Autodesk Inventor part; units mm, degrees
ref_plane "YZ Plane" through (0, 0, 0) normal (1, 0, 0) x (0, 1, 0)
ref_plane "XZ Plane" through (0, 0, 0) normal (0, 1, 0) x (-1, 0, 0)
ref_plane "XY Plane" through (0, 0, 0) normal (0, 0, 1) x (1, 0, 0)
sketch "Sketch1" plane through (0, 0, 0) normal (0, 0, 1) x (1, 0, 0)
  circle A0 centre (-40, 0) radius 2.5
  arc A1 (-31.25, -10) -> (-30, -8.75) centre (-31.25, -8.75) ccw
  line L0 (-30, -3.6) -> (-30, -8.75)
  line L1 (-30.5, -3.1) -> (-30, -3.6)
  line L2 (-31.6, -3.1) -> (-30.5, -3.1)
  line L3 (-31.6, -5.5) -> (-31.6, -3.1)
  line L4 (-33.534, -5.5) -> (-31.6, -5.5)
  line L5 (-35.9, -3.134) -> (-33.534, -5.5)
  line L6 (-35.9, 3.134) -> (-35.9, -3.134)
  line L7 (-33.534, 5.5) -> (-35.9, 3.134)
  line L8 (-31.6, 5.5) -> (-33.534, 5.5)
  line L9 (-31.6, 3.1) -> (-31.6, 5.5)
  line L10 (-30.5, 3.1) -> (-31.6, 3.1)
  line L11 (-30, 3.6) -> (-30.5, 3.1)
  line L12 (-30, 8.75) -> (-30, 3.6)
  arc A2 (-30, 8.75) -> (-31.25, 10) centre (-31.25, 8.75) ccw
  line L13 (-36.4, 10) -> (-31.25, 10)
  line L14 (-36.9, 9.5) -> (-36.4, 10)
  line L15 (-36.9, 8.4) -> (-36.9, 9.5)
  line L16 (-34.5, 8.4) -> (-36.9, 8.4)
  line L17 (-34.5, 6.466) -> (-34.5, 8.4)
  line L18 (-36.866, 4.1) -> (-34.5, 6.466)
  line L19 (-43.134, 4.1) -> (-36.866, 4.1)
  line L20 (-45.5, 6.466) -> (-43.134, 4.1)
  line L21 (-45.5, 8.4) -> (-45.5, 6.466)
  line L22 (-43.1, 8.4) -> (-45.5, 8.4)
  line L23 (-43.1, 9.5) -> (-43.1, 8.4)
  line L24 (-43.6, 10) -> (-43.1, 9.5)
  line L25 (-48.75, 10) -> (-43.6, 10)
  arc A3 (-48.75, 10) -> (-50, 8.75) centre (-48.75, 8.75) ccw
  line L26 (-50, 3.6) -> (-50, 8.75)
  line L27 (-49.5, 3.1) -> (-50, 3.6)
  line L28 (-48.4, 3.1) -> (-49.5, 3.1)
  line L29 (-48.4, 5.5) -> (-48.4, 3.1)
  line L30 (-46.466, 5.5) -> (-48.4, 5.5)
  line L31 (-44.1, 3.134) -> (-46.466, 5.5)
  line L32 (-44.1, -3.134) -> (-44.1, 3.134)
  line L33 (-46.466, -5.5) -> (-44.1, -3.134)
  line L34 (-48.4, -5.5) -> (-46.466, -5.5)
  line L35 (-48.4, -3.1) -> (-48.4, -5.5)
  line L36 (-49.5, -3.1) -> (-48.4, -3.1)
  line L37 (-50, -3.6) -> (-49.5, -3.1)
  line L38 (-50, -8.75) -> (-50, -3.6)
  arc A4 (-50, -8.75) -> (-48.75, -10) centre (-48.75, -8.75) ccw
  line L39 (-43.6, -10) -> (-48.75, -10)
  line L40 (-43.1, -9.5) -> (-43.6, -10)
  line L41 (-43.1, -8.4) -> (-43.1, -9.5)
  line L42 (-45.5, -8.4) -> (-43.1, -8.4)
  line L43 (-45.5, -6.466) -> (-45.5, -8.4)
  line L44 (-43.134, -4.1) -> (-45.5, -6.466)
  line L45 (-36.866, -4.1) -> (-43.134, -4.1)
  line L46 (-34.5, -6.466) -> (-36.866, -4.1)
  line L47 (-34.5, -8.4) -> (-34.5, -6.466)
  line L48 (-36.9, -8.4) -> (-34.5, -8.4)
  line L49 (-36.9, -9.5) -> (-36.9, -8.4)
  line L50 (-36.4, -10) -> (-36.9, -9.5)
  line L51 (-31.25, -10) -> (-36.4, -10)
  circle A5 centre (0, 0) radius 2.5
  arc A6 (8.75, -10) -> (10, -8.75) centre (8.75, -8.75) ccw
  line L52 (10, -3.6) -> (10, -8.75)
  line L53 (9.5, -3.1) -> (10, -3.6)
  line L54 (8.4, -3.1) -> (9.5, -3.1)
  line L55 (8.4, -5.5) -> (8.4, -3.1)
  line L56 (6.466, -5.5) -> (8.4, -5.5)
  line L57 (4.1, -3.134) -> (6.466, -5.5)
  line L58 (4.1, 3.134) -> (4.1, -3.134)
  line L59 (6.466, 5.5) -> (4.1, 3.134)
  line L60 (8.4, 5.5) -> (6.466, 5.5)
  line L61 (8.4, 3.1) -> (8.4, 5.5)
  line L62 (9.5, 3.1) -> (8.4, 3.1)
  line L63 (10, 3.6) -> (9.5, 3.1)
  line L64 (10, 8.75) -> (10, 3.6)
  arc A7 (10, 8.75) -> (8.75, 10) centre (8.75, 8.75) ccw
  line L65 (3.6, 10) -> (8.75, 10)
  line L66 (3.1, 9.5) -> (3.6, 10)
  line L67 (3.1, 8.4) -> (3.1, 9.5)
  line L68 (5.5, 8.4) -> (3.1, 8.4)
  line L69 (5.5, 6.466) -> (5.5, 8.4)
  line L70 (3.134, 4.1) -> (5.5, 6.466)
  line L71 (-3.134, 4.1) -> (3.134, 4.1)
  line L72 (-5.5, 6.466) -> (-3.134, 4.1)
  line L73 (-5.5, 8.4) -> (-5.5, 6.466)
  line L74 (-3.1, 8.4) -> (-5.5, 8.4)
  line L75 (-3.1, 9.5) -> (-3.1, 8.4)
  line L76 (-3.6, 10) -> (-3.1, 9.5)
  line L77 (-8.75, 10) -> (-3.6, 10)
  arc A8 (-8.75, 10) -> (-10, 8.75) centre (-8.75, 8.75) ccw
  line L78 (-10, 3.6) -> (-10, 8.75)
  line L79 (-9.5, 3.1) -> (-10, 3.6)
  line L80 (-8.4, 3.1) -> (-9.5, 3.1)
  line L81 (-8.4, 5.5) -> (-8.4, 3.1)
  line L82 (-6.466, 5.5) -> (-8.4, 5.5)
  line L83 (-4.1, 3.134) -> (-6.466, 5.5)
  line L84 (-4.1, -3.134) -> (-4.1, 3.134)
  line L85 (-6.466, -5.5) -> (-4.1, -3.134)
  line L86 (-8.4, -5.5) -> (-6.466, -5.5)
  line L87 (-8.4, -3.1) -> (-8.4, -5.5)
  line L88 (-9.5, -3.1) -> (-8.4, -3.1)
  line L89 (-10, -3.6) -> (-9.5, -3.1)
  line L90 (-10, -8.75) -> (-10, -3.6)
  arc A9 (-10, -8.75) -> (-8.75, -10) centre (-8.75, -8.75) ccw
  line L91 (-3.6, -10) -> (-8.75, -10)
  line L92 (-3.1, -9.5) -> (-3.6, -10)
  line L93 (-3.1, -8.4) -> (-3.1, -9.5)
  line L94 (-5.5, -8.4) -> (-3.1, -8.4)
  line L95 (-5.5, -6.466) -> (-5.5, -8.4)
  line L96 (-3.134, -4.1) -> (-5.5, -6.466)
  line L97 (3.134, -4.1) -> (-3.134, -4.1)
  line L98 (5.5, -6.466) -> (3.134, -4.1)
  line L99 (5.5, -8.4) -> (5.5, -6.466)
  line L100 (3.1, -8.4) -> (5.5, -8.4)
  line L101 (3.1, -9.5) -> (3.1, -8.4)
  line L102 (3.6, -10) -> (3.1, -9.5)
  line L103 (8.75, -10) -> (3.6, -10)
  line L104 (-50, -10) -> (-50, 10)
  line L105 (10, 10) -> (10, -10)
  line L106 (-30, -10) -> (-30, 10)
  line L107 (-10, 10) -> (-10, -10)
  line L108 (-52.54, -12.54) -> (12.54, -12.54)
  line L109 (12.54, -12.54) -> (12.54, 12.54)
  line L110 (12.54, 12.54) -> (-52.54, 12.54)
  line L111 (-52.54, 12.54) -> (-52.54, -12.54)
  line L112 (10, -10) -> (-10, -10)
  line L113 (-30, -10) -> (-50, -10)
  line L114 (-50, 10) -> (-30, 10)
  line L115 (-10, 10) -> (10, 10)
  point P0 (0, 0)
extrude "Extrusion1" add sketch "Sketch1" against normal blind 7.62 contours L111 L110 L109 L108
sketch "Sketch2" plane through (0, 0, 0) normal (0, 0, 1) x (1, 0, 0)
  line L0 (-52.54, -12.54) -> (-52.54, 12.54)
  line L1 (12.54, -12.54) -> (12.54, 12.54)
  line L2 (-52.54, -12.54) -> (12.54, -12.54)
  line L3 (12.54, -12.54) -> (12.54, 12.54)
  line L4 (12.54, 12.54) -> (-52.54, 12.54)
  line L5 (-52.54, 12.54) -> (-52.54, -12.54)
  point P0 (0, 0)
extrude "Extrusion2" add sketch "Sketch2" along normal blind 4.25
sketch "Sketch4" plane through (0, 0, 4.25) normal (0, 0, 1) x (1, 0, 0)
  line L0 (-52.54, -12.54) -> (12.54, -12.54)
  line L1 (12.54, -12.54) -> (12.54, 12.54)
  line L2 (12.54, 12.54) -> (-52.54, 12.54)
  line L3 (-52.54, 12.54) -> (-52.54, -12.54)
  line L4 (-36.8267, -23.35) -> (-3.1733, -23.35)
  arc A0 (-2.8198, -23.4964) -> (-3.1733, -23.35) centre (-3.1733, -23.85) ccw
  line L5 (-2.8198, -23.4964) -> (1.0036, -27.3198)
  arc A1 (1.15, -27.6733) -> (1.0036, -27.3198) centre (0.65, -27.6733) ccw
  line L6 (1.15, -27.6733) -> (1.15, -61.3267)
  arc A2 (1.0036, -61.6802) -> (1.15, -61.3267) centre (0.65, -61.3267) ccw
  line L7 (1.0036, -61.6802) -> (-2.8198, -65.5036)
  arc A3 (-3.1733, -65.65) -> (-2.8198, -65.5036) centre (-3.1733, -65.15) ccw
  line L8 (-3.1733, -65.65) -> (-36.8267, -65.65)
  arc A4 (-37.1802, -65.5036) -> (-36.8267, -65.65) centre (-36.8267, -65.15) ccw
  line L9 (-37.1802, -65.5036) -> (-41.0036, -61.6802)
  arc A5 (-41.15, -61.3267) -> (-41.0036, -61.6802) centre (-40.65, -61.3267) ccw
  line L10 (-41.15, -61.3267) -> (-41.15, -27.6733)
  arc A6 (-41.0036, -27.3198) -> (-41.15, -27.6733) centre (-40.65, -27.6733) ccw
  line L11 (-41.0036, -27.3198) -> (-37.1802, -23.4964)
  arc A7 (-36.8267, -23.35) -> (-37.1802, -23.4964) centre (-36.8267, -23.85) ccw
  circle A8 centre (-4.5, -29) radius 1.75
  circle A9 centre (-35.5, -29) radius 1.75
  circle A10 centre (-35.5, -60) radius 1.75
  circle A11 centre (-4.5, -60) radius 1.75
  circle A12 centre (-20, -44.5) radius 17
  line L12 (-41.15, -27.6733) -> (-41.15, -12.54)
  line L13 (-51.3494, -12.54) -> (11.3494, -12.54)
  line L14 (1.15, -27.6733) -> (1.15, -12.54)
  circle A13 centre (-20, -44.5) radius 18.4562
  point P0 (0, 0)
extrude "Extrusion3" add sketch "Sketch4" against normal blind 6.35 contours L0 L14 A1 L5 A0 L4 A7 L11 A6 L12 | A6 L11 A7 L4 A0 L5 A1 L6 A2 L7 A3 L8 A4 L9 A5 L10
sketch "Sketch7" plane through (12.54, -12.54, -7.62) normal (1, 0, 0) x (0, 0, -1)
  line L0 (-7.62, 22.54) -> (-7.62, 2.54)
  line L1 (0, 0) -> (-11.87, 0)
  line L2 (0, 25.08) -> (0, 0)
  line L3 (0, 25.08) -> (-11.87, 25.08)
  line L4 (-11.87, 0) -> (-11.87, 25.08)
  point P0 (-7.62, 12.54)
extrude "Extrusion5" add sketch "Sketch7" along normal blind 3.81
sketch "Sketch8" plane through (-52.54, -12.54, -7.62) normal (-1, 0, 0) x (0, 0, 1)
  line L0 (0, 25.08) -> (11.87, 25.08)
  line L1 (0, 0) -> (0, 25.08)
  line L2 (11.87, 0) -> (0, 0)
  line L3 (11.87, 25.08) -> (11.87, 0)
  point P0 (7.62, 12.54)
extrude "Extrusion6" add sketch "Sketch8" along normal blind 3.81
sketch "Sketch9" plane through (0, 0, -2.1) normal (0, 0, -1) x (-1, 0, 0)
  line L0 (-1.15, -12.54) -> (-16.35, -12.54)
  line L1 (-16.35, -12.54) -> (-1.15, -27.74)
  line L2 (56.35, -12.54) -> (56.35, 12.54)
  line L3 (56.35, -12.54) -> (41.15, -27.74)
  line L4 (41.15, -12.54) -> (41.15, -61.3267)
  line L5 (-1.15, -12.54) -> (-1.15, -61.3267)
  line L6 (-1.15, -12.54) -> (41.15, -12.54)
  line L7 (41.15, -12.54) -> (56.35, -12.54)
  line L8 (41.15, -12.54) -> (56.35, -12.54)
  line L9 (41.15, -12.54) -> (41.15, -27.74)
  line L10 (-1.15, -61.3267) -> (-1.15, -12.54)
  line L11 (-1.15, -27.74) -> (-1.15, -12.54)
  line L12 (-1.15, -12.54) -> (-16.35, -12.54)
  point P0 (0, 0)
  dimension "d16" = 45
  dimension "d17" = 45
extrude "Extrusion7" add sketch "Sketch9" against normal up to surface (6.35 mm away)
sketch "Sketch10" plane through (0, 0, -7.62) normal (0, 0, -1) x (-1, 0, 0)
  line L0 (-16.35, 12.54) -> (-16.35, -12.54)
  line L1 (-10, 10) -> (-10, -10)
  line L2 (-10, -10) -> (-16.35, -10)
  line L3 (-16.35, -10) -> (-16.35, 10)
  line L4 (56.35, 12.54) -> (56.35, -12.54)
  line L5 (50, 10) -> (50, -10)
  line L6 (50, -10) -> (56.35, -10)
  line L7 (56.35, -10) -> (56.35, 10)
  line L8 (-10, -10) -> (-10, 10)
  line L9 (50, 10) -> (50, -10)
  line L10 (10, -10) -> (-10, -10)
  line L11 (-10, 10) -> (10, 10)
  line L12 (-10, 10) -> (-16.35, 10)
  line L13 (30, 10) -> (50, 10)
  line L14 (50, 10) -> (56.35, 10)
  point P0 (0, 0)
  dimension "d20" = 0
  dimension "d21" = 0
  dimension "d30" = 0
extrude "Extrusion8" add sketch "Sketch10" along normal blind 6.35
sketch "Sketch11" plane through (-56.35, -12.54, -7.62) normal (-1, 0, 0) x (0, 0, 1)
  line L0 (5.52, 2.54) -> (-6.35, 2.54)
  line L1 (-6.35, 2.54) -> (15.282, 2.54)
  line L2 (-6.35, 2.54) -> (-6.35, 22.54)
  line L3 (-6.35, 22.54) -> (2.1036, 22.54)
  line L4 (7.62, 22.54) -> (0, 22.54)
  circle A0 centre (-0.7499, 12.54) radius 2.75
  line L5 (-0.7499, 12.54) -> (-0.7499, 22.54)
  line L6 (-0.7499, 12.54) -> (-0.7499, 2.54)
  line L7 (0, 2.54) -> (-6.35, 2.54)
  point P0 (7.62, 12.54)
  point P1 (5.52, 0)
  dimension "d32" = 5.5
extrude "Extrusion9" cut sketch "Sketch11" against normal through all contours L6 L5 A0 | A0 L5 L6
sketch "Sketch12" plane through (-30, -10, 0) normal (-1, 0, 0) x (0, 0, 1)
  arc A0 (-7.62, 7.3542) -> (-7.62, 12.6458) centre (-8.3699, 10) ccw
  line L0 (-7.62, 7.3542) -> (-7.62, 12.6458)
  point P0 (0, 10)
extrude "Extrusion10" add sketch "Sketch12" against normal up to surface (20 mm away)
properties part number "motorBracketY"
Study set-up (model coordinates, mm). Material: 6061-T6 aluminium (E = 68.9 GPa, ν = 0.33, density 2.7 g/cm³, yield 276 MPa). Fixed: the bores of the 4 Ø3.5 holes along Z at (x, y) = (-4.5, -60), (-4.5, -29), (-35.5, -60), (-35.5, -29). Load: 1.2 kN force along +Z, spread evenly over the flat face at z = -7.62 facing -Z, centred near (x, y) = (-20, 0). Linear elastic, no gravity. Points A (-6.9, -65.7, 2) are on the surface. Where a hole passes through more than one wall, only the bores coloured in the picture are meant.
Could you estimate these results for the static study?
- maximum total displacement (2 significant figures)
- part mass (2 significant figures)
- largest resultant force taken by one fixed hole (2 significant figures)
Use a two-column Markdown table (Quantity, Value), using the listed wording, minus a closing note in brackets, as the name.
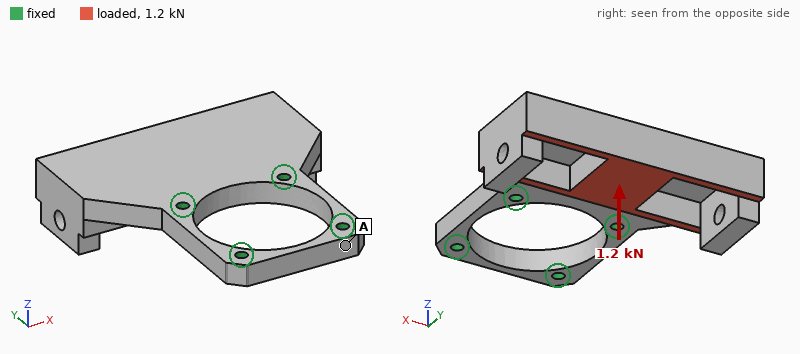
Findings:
| Quantity | Value |
|---|---|
| maximum total displacement | 0.33 mm |
| part mass | 69 g |
| largest resultant force taken by one fixed hole | 630 N |
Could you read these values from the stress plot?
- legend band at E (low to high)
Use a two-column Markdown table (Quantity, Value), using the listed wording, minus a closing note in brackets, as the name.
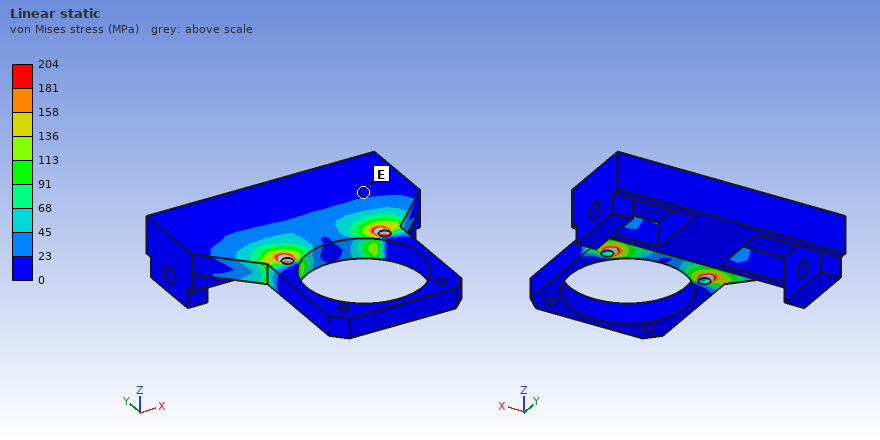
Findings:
| Quantity | Value |
|---|---|
| legend band at E | 0 to 23 MPa |
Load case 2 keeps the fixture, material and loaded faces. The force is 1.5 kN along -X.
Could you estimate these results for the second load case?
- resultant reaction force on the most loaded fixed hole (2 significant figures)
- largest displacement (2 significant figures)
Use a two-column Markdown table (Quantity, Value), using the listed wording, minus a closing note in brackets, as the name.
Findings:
| Quantity | Value |
|---|---|
| resultant reaction force on the most loaded fixed hole | 1.5 kN |
| largest displacement | 63 µm |
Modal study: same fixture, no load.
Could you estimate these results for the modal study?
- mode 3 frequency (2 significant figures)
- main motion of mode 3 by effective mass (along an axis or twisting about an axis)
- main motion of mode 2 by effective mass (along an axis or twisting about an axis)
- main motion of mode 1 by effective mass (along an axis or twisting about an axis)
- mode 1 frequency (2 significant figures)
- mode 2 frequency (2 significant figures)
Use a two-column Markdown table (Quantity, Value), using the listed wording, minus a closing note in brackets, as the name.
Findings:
| Quantity | Value |
|---|---|
| mode 3 frequency | 6900 Hz |
| main motion of mode 3 by effective mass | along X |
| main motion of mode 2 by effective mass | twisting about Y |
| main motion of mode 1 by effective mass | along Z |
| mode 1 frequency | 1700 Hz |
| mode 2 frequency | 3100 Hz |
